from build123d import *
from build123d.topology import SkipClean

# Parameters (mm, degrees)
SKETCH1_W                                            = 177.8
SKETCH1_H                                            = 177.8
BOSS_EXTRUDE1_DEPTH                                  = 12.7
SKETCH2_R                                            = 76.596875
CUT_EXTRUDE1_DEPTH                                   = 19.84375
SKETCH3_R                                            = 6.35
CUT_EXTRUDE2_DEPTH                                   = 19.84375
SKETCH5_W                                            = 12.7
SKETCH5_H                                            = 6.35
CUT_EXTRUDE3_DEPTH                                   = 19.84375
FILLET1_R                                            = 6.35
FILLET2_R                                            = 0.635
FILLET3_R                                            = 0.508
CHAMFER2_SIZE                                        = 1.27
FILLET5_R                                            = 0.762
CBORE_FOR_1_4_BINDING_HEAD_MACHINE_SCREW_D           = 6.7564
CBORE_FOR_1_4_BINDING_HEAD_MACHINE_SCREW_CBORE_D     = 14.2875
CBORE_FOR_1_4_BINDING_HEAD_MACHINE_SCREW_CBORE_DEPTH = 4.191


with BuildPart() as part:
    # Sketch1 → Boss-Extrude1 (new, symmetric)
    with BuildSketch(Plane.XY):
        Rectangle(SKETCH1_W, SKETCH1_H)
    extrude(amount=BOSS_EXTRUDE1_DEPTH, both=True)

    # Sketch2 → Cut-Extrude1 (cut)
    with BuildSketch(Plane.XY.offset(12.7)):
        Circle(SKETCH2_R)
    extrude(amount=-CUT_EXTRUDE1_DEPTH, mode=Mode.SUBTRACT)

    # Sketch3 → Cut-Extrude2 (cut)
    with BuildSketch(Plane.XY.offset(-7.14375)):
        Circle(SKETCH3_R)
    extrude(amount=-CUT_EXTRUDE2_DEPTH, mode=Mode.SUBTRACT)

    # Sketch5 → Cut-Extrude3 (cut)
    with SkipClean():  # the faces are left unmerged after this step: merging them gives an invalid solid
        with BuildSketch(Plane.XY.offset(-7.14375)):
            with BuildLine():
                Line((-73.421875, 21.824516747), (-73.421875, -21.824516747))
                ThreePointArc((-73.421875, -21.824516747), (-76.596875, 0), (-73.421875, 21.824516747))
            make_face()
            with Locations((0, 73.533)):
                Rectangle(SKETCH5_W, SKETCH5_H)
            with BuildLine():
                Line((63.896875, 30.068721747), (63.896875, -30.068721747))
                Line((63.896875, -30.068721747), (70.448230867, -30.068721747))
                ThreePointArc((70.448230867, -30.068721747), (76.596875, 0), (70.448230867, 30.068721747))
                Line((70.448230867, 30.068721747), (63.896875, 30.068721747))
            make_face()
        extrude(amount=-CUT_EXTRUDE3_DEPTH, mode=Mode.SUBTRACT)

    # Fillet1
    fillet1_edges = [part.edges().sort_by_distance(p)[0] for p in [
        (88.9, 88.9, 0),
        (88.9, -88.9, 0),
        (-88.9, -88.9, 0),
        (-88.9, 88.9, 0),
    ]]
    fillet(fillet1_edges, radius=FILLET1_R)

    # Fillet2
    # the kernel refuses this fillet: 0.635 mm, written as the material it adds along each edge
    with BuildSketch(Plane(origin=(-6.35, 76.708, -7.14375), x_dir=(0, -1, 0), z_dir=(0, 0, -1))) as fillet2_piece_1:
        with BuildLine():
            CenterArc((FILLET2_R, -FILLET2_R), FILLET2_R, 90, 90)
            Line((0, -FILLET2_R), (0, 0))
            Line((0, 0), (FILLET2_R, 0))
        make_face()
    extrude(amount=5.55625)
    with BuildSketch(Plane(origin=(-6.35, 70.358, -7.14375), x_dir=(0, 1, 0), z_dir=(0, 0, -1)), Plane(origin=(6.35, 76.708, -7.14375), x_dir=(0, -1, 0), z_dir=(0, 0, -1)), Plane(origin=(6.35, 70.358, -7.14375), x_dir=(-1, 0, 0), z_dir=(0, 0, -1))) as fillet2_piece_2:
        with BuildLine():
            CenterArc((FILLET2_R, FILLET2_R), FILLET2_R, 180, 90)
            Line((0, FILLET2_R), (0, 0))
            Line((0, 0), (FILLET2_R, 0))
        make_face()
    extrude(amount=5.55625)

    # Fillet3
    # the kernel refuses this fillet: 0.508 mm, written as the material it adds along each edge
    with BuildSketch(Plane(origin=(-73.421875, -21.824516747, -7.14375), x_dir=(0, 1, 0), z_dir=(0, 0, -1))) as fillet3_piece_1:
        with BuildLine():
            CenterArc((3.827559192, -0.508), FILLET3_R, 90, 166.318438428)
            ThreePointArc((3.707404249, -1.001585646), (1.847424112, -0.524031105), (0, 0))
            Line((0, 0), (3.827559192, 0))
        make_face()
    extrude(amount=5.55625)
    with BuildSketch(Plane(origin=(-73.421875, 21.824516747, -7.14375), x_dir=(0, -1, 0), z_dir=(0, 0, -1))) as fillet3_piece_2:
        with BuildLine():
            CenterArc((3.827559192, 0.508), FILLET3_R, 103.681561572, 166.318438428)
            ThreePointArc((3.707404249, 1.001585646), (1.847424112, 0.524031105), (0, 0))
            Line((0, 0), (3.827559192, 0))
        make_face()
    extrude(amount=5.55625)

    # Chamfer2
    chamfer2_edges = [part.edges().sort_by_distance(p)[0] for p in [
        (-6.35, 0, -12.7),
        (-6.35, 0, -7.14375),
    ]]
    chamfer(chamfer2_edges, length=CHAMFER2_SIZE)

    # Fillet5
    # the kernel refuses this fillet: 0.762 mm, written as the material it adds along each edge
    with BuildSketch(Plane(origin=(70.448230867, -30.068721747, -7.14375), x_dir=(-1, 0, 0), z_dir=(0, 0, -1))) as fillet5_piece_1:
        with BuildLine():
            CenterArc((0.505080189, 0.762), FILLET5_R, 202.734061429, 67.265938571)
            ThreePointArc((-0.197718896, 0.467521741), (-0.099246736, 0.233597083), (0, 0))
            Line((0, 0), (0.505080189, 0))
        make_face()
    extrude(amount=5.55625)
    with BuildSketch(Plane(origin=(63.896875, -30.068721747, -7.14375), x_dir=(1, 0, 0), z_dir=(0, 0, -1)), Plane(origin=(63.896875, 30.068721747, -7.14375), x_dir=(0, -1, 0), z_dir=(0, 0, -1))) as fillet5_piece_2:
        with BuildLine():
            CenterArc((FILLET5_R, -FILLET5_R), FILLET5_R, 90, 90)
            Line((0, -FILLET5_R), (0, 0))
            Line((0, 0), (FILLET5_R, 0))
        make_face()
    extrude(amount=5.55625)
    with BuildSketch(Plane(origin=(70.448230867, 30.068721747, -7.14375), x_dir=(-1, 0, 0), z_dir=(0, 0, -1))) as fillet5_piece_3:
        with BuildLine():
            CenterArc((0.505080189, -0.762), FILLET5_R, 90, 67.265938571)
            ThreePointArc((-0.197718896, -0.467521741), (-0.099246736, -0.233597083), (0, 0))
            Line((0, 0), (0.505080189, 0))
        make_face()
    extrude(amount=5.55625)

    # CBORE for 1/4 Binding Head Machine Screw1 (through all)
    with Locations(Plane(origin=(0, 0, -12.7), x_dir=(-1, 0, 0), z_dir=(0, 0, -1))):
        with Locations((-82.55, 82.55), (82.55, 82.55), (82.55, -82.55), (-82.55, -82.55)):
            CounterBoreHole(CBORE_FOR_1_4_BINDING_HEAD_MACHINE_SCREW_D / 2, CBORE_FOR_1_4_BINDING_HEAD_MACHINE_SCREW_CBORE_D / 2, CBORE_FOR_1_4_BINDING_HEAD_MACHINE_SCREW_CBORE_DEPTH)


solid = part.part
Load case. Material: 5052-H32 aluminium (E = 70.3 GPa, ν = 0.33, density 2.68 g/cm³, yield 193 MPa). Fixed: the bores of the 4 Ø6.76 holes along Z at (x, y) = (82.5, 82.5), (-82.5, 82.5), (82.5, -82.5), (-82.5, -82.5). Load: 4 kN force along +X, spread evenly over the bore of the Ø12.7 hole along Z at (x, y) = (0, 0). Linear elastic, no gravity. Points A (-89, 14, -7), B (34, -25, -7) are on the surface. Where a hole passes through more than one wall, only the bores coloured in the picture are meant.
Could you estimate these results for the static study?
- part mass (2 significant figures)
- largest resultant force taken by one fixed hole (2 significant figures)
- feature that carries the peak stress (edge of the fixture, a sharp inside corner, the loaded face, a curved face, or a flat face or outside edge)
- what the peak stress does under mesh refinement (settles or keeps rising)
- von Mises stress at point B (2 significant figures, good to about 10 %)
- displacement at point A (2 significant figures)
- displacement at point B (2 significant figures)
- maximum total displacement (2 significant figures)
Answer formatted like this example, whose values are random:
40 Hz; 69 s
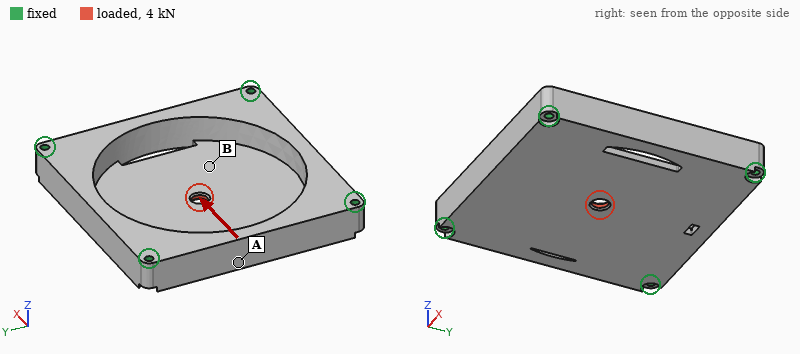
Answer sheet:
1.1 kg; 1.1 kN; a sharp inside corner; keeps rising; 5.9 MPa; 4.7 µm; 6.4 µm; 11 µm
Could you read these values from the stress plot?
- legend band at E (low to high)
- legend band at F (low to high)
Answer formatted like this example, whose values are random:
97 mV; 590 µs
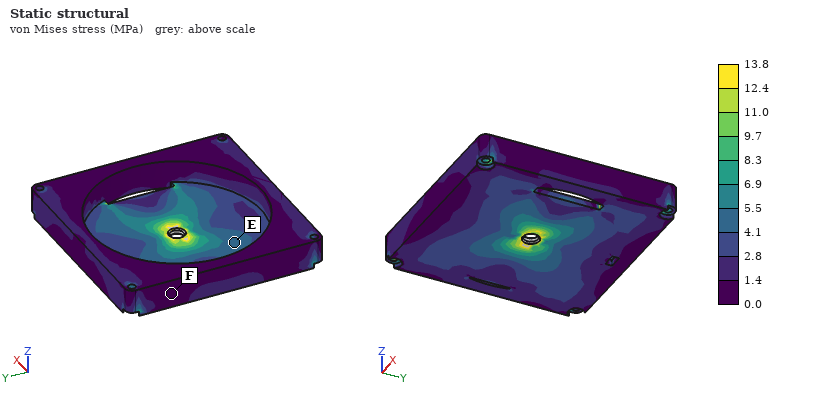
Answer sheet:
4.1 to 5.5 MPa; 0.0 to 1.4 MPa
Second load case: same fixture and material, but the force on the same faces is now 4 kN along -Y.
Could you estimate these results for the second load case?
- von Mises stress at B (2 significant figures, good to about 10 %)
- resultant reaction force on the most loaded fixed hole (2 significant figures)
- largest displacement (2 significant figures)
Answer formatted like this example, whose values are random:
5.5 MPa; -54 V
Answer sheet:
5.0 MPa; 1.2 kN; 11 µm
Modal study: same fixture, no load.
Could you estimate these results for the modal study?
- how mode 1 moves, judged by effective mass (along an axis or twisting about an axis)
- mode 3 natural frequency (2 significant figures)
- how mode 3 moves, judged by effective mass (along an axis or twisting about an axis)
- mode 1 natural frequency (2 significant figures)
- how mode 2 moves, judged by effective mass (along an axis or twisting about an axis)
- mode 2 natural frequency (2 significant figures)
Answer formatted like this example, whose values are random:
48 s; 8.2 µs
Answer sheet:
along Z; 3400 Hz; twisting about X; 1900 Hz; twisting about Y; 3200 Hz
